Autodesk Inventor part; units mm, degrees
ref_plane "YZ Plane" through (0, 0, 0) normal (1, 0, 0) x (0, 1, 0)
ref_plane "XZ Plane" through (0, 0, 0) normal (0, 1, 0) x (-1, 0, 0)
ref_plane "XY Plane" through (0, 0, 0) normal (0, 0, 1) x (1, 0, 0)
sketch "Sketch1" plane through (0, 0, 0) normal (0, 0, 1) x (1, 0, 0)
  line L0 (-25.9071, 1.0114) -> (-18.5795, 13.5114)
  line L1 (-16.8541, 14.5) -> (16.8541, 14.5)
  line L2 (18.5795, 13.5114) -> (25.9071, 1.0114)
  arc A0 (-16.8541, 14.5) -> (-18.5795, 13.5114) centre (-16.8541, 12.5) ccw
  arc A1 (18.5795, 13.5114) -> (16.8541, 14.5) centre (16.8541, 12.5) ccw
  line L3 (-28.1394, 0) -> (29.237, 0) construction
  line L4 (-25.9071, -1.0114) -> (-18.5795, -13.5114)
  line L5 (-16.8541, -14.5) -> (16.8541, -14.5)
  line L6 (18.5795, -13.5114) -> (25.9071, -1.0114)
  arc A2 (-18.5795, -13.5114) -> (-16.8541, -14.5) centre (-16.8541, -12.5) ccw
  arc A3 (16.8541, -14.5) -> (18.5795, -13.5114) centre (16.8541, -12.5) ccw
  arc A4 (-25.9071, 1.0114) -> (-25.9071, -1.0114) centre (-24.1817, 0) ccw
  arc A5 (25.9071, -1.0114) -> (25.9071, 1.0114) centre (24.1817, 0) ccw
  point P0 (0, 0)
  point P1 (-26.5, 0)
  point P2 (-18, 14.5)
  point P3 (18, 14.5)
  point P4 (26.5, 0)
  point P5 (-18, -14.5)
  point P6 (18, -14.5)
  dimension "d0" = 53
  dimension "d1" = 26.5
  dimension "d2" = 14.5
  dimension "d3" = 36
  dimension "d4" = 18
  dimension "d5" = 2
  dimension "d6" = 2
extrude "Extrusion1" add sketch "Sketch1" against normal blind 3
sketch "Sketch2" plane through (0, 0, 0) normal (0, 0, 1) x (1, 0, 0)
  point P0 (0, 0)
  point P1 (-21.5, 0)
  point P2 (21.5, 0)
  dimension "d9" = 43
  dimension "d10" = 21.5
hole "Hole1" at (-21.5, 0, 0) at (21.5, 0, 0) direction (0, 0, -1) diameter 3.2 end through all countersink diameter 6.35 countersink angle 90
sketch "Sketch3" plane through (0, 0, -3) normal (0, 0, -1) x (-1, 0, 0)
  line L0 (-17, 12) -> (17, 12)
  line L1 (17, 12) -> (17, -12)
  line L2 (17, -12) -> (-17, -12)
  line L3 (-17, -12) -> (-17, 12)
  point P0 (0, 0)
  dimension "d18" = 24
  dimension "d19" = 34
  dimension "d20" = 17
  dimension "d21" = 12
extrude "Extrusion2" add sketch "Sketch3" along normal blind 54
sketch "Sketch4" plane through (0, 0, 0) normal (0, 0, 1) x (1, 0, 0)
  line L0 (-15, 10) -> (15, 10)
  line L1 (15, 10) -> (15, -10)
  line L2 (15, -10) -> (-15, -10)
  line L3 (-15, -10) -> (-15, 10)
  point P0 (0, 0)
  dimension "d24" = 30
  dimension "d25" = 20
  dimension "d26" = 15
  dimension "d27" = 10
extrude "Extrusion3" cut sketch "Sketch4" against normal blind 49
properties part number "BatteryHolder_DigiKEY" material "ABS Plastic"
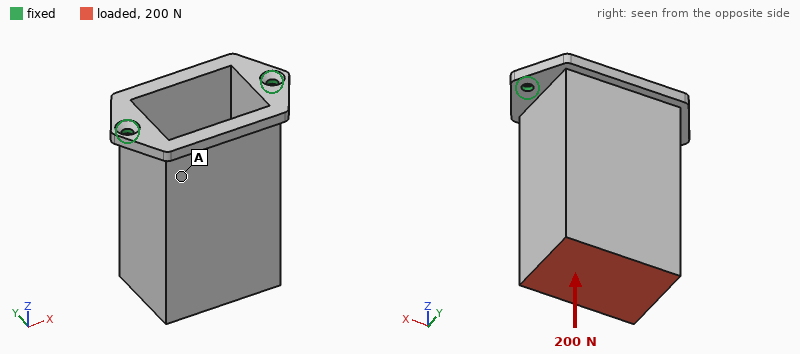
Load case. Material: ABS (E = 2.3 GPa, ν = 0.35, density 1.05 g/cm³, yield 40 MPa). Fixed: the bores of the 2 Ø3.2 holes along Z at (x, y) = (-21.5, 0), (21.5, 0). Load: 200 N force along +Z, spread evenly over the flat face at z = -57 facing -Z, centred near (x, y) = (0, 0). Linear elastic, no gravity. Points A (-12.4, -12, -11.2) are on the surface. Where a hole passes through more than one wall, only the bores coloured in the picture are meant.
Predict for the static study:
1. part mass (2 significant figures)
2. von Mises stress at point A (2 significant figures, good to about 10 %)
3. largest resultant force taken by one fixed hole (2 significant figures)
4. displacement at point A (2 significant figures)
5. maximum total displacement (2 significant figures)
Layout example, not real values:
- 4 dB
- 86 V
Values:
- 19 g
- 1.8 MPa
- 100 N
- 0.12 mm
- 0.14 mm
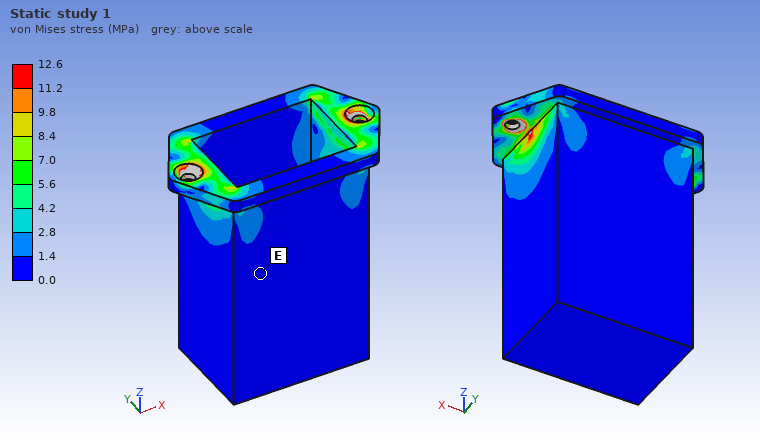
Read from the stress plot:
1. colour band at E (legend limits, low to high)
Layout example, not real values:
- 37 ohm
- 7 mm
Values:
- 0.0 to 1.4 MPa
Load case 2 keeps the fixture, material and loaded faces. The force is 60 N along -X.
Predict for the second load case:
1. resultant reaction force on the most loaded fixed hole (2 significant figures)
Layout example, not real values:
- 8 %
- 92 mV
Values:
- 92 N
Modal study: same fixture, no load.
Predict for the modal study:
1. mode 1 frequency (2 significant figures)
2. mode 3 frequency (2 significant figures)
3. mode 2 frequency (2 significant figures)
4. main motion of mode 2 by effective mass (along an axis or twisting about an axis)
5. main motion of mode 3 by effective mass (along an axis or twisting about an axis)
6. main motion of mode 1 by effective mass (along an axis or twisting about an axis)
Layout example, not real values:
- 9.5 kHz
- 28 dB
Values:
- 160 Hz
- 1400 Hz
- 680 Hz
- along X
- along Z
- along Y
